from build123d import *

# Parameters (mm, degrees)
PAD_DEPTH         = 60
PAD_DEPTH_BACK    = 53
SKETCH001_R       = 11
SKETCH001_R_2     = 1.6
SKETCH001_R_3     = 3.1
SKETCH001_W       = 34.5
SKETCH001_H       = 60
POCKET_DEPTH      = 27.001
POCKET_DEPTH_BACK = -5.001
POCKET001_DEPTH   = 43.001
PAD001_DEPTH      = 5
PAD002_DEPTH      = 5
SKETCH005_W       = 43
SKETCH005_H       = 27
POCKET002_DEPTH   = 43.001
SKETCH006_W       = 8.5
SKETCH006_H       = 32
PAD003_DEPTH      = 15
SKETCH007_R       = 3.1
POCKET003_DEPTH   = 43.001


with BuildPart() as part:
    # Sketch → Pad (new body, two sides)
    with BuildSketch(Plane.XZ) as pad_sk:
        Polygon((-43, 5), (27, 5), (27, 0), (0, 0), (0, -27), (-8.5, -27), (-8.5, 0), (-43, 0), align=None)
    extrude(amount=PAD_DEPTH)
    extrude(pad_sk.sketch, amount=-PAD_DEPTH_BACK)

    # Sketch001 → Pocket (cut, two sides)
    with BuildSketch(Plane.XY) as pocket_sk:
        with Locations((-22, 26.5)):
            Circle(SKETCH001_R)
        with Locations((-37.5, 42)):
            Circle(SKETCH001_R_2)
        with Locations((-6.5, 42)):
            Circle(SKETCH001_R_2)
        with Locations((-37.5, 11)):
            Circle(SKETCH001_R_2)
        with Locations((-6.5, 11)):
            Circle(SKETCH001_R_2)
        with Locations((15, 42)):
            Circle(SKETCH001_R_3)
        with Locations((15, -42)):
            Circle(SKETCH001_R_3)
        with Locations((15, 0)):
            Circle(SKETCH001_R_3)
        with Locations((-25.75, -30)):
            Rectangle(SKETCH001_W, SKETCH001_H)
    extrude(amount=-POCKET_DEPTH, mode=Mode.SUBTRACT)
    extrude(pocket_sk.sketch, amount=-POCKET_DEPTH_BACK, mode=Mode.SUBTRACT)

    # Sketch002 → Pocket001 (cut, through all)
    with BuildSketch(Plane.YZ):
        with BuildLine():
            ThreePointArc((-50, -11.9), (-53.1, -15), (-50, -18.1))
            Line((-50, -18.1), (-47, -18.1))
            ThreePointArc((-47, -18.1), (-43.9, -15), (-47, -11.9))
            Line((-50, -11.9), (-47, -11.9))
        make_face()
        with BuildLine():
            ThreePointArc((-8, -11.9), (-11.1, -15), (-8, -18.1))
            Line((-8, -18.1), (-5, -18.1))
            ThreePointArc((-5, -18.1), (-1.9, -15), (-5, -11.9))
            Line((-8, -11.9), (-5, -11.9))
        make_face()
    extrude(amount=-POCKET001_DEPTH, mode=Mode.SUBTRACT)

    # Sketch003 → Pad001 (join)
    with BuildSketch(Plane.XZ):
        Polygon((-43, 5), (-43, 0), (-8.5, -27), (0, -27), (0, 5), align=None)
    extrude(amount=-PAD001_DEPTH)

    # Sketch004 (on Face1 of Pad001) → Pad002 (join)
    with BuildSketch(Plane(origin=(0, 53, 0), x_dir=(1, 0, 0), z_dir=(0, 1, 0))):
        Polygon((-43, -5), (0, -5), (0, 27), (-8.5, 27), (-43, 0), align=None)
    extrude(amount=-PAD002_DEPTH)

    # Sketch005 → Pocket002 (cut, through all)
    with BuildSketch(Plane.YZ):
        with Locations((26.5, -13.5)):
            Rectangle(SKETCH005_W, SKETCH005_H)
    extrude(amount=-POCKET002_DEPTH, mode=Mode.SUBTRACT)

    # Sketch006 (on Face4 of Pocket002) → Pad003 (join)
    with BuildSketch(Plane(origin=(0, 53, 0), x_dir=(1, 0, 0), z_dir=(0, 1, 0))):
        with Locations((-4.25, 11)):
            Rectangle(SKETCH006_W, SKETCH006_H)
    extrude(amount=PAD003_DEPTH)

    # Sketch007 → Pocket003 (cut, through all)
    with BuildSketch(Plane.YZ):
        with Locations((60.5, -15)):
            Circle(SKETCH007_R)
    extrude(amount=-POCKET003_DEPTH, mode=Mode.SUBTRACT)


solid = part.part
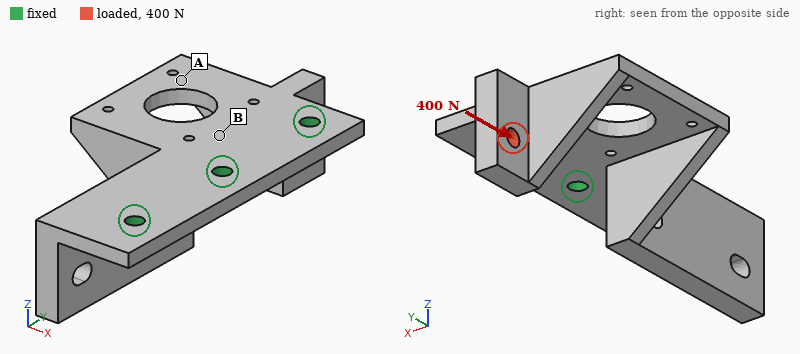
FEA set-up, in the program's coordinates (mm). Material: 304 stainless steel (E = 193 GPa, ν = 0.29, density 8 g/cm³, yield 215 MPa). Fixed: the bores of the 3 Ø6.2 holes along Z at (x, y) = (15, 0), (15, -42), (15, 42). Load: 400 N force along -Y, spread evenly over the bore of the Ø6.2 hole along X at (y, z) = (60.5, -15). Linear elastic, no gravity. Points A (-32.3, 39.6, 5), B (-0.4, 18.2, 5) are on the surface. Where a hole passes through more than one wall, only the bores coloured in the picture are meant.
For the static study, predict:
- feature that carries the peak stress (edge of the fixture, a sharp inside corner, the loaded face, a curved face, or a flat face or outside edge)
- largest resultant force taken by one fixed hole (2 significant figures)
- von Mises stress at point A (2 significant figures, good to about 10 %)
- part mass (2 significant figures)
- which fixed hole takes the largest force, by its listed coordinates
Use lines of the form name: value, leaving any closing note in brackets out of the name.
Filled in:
feature that carries the peak stress: a curved face
largest resultant force taken by one fixed hole: 270 N
von Mises stress at point A: 15 MPa
part mass: 400 g
which fixed hole takes the largest force, by its listed coordinates: (15, 42)
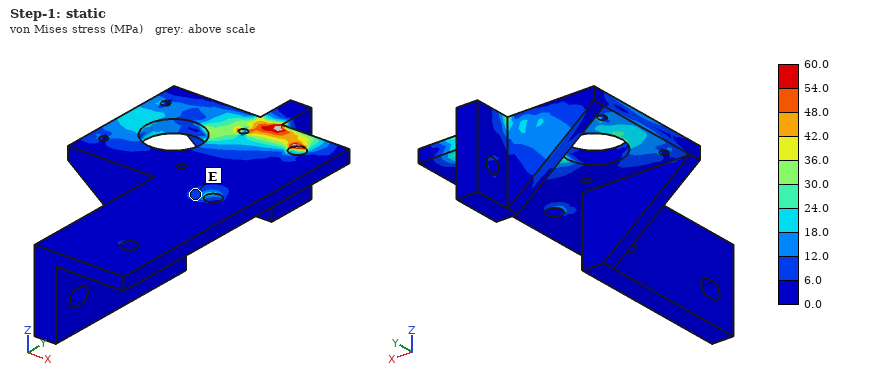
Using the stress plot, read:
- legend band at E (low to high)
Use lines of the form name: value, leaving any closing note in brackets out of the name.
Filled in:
legend band at E: 6.0 to 12.0 MPa
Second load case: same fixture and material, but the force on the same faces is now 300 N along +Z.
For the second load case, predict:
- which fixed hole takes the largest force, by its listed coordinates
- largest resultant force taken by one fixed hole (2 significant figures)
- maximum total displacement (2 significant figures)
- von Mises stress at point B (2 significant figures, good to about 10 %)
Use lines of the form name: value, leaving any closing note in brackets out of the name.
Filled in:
which fixed hole takes the largest force, by its listed coordinates: (15, 42)
largest resultant force taken by one fixed hole: 360 N
maximum total displacement: 63 µm
von Mises stress at point B: 6.6 MPa
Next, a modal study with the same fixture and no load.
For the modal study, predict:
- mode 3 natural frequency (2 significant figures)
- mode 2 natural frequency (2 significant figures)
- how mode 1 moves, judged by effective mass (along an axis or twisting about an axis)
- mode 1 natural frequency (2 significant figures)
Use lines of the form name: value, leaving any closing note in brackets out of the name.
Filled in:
mode 3 natural frequency: 2700 Hz
mode 2 natural frequency: 1700 Hz
how mode 1 moves, judged by effective mass: along Z
mode 1 natural frequency: 1200 Hz
